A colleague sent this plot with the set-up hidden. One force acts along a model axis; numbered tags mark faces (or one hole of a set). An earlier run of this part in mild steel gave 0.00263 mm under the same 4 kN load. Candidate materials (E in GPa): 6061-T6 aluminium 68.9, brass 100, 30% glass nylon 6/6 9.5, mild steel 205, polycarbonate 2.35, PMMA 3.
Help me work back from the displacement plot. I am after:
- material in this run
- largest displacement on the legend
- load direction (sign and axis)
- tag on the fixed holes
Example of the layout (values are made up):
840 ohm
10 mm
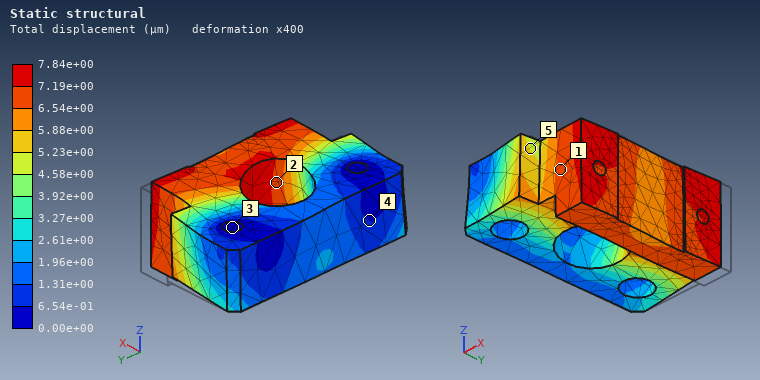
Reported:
6061-T6 aluminium
7.84e+00 µm
-Y
3
